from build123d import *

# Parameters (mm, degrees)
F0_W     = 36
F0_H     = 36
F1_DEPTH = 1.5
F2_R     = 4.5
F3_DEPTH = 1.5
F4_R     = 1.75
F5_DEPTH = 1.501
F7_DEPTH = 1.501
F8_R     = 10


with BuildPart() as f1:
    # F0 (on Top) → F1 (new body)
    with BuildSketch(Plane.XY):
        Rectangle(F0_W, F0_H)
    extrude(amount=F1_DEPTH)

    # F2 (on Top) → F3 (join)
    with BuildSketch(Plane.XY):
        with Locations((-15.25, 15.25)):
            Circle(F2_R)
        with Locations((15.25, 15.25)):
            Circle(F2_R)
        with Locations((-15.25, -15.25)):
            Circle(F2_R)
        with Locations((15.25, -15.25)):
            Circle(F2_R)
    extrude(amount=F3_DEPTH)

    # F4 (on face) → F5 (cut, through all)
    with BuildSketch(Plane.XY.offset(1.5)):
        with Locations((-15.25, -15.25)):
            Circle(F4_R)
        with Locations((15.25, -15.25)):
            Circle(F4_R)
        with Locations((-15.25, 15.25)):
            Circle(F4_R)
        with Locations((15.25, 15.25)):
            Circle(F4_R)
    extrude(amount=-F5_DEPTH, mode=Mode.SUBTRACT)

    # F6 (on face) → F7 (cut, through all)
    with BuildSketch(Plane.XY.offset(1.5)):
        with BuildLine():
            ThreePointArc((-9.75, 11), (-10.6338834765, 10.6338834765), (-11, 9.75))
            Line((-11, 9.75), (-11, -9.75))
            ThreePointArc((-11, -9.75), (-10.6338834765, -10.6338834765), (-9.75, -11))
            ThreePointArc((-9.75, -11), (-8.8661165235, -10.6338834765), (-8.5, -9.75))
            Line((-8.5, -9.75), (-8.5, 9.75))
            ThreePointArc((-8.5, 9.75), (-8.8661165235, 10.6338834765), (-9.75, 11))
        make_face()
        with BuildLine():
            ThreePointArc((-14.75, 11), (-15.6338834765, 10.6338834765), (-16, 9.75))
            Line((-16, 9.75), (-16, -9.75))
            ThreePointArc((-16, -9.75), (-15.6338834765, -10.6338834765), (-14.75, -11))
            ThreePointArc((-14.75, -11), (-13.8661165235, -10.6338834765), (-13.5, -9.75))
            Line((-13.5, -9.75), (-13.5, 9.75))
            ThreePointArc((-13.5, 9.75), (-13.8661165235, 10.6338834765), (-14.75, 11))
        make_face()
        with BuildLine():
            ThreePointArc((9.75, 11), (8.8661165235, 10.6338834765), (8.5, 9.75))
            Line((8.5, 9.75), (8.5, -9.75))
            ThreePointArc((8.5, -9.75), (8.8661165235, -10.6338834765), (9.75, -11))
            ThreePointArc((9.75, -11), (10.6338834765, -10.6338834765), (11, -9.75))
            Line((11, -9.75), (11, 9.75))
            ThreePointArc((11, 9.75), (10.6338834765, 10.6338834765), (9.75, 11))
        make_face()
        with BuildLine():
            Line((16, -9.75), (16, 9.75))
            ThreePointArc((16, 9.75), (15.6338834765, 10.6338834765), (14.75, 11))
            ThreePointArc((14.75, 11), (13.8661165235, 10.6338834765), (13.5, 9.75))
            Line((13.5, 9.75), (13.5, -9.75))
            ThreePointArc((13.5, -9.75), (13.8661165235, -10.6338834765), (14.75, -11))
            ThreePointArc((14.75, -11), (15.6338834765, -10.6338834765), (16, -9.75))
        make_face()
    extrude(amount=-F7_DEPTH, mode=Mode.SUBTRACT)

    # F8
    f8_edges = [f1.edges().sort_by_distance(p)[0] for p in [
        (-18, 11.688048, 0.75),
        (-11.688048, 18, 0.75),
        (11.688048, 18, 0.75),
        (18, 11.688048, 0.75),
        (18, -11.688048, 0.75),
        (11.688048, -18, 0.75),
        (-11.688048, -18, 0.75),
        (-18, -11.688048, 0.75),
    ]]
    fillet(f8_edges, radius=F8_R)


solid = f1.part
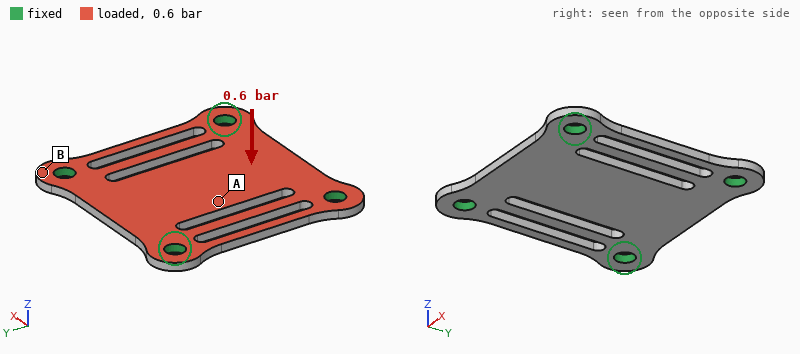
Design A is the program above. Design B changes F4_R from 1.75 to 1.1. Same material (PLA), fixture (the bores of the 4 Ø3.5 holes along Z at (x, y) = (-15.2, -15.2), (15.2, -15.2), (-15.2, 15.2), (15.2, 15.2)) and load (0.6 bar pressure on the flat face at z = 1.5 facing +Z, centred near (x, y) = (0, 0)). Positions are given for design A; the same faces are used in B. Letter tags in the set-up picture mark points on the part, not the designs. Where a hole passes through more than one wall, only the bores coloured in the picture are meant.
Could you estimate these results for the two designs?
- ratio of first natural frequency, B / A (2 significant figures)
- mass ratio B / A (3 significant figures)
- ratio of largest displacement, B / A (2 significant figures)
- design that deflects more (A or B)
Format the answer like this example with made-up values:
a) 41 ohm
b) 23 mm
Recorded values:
a) 0.93
b) 1.02
c) 1.2
d) B
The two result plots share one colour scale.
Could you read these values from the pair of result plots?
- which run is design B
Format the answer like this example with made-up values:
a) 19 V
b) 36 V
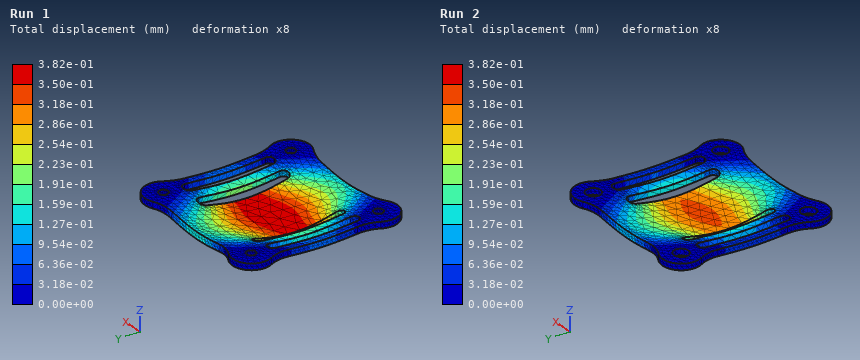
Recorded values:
a) Run 1
